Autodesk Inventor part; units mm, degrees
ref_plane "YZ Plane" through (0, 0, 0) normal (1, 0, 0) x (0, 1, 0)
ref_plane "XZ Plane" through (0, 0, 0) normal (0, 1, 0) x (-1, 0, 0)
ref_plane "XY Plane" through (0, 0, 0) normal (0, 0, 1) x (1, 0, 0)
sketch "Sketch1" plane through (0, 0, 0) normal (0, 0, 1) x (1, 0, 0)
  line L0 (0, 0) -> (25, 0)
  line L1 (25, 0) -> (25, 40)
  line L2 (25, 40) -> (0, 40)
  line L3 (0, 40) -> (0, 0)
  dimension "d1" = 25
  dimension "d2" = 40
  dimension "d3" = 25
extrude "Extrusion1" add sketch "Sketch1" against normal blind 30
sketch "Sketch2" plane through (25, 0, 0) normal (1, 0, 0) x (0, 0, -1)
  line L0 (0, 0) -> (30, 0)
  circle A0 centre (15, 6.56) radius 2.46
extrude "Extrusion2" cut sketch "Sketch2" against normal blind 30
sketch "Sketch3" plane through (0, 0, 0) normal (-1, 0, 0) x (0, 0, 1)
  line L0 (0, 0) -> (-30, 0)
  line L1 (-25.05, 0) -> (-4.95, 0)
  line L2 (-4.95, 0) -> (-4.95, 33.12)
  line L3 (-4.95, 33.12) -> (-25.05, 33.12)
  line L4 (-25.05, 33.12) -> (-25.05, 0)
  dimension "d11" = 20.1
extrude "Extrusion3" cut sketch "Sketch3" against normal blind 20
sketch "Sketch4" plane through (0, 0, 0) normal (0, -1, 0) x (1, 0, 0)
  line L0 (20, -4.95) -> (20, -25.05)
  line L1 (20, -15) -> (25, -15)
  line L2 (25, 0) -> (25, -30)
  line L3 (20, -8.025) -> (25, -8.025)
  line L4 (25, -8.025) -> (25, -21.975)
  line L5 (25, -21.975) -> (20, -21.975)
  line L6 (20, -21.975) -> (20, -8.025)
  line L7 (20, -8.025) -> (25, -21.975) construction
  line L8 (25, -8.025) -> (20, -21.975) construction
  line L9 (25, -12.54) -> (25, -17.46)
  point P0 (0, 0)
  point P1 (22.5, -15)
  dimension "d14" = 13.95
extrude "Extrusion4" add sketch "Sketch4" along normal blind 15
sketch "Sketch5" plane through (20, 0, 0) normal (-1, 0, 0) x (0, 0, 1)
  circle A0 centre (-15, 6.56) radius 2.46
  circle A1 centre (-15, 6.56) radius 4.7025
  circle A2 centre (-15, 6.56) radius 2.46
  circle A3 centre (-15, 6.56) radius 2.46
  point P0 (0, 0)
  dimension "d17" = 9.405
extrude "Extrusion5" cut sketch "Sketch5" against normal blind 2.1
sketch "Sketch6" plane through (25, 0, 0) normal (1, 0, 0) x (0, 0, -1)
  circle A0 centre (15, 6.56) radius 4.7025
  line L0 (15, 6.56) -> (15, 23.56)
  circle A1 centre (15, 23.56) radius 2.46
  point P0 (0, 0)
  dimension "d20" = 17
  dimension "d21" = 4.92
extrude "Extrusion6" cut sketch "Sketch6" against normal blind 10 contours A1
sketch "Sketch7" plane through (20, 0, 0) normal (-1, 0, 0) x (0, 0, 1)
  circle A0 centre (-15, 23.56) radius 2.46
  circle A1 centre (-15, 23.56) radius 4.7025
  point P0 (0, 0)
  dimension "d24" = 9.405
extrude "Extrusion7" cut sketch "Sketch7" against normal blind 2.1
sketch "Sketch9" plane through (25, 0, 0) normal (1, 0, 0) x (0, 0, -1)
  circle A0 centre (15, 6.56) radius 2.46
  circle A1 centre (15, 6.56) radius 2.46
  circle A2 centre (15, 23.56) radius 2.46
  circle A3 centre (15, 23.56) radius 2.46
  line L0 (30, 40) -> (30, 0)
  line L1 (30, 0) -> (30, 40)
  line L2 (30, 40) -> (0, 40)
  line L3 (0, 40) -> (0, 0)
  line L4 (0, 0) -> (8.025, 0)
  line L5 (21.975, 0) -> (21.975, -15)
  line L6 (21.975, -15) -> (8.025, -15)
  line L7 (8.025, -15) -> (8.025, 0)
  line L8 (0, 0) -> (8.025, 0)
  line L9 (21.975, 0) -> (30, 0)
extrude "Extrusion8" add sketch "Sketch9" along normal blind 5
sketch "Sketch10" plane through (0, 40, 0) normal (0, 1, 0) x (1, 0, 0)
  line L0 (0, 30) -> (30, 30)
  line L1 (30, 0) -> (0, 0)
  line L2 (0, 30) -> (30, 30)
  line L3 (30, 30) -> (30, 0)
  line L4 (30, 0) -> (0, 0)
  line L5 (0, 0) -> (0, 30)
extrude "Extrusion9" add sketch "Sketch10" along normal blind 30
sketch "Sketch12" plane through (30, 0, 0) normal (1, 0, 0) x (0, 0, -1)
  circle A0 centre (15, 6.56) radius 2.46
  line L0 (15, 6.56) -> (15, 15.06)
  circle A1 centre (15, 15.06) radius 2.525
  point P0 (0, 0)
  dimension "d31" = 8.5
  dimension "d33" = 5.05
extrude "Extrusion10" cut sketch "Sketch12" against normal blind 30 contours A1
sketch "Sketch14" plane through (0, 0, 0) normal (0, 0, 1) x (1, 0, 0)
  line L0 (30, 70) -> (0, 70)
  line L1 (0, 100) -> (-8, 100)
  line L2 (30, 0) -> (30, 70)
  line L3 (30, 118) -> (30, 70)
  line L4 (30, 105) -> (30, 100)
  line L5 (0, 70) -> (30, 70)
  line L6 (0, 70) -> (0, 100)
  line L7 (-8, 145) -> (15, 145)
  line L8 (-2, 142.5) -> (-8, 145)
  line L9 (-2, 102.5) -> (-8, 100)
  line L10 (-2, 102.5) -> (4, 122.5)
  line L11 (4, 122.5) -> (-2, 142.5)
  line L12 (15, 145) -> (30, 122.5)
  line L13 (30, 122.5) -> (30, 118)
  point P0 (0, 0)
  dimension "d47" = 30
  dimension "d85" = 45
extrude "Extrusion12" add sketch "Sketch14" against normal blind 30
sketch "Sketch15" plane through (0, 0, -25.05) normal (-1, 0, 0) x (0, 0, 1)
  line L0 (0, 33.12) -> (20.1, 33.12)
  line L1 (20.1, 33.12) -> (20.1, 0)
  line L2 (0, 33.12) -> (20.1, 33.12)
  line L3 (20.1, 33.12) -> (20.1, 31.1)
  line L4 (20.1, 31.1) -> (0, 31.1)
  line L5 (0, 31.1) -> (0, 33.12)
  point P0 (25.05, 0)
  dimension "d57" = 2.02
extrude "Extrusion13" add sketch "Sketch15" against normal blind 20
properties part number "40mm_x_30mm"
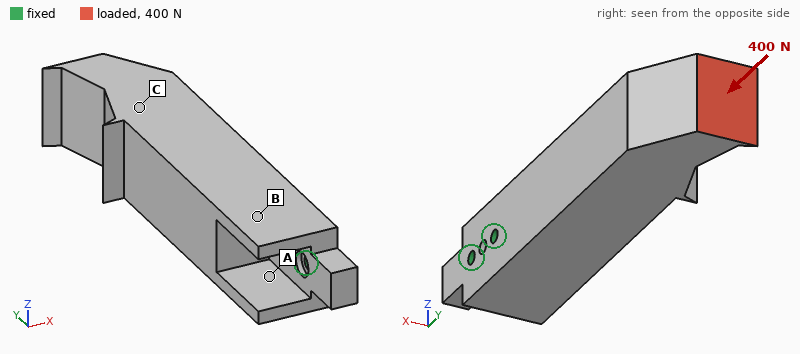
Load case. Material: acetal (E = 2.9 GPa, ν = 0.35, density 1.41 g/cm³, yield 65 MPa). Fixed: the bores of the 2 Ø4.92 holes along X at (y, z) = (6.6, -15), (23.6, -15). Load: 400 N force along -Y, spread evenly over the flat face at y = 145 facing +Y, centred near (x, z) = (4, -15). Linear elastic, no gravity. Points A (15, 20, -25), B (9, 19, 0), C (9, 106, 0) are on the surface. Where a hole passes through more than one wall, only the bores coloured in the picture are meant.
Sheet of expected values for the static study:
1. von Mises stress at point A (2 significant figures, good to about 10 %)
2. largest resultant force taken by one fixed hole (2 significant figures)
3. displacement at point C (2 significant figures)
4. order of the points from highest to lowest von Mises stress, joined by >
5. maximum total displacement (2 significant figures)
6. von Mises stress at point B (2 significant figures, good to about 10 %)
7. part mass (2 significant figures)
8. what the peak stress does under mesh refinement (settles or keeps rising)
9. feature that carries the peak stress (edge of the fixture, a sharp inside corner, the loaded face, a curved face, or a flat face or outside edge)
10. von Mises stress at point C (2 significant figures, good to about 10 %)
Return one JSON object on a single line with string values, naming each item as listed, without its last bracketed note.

{"von Mises stress at point A": "3.4 MPa", "largest resultant force taken by one fixed hole": "410 N", "displacement at point C": "0.45 mm", "order of the points from highest to lowest von Mises stress, joined by >": "A > B > C", "maximum total displacement": "0.83 mm", "von Mises stress at point B": "2.4 MPa", "part mass": "160 g", "what the peak stress does under mesh refinement": "keeps rising", "feature that carries the peak stress": "edge of the fixture", "von Mises stress at point C": "1.1 MPa"}
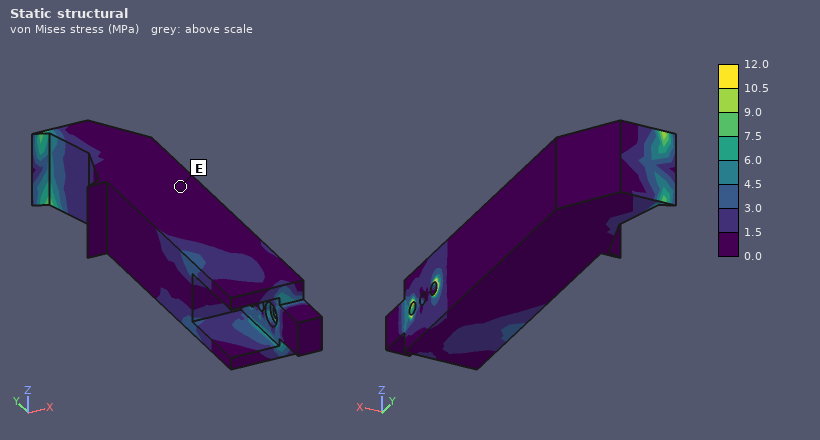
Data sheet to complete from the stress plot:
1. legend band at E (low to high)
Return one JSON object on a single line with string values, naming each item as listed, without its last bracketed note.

{"legend band at E": "0.0 to 1.5 MPa"}
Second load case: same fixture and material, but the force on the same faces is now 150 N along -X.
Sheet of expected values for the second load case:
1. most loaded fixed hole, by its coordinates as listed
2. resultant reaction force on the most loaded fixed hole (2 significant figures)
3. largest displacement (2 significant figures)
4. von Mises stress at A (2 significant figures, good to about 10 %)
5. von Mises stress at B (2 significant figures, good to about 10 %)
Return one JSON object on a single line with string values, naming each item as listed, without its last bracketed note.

{"most loaded fixed hole, by its coordinates as listed": "(23.6, -15)", "resultant reaction force on the most loaded fixed hole": "880 N", "largest displacement": "1.7 mm", "von Mises stress at A": "6.5 MPa", "von Mises stress at B": "4.9 MPa"}
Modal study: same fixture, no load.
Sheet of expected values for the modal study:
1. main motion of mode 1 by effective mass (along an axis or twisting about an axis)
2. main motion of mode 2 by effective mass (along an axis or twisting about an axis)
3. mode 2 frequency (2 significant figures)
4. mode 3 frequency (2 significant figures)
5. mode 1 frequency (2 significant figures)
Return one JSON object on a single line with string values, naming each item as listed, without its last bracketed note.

{"main motion of mode 1 by effective mass": "along X", "main motion of mode 2 by effective mass": "along Z", "mode 2 frequency": "280 Hz", "mode 3 frequency": "850 Hz", "mode 1 frequency": "240 Hz"}
